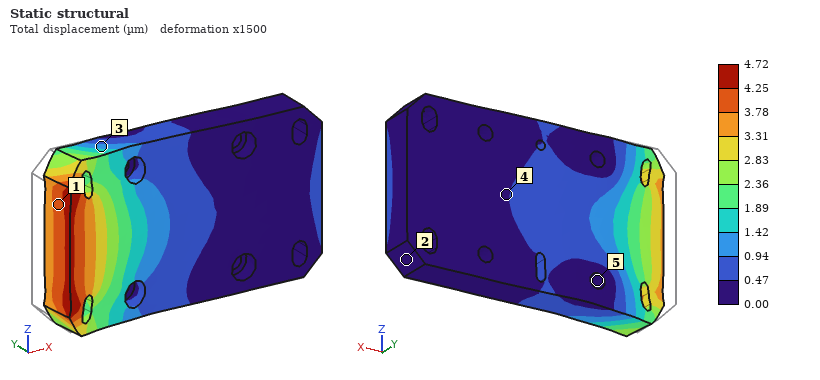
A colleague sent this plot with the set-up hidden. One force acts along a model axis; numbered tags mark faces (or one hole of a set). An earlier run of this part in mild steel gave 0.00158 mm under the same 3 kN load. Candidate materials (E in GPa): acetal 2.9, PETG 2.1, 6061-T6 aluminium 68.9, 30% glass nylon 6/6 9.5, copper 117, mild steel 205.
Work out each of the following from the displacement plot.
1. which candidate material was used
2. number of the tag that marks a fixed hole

6061-T6 aluminium
5
